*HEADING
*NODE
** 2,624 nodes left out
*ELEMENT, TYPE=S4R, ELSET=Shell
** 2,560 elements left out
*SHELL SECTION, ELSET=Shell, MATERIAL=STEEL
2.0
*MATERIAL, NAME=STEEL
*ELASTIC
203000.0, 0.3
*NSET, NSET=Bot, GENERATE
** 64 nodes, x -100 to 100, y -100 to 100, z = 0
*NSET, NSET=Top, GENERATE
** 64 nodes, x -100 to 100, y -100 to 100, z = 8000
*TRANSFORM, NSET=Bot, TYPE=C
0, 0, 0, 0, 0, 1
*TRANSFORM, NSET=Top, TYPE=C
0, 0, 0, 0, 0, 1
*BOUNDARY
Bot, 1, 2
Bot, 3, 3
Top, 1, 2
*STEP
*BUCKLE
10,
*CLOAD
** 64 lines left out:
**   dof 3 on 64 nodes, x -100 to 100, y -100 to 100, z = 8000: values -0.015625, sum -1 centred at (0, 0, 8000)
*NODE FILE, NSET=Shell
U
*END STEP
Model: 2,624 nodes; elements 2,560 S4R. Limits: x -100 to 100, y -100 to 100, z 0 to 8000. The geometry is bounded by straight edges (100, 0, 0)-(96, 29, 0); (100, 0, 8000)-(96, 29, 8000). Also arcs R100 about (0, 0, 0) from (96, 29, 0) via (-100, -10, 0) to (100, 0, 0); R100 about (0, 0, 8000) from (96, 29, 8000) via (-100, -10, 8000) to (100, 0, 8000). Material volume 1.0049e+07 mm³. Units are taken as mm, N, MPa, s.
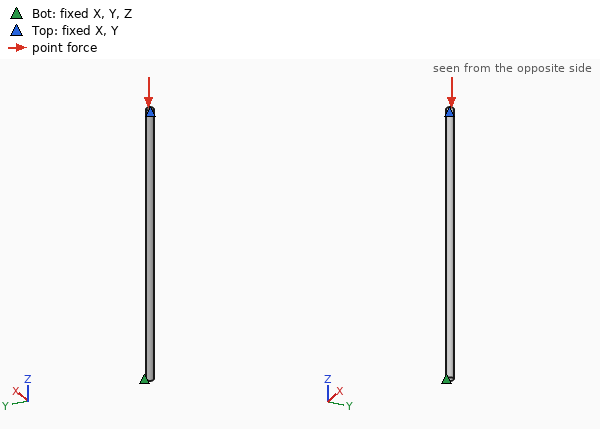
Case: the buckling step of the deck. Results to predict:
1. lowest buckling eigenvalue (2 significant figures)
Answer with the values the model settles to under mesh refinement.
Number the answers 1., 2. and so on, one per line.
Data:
1. 4.0e+05
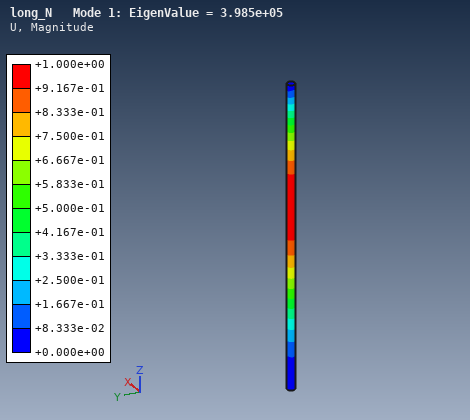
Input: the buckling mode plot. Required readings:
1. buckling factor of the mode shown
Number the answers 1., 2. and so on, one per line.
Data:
1. 3.985e+05
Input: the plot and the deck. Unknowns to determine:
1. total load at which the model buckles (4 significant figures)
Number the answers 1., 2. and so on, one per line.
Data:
1. 3.985e+05 N
